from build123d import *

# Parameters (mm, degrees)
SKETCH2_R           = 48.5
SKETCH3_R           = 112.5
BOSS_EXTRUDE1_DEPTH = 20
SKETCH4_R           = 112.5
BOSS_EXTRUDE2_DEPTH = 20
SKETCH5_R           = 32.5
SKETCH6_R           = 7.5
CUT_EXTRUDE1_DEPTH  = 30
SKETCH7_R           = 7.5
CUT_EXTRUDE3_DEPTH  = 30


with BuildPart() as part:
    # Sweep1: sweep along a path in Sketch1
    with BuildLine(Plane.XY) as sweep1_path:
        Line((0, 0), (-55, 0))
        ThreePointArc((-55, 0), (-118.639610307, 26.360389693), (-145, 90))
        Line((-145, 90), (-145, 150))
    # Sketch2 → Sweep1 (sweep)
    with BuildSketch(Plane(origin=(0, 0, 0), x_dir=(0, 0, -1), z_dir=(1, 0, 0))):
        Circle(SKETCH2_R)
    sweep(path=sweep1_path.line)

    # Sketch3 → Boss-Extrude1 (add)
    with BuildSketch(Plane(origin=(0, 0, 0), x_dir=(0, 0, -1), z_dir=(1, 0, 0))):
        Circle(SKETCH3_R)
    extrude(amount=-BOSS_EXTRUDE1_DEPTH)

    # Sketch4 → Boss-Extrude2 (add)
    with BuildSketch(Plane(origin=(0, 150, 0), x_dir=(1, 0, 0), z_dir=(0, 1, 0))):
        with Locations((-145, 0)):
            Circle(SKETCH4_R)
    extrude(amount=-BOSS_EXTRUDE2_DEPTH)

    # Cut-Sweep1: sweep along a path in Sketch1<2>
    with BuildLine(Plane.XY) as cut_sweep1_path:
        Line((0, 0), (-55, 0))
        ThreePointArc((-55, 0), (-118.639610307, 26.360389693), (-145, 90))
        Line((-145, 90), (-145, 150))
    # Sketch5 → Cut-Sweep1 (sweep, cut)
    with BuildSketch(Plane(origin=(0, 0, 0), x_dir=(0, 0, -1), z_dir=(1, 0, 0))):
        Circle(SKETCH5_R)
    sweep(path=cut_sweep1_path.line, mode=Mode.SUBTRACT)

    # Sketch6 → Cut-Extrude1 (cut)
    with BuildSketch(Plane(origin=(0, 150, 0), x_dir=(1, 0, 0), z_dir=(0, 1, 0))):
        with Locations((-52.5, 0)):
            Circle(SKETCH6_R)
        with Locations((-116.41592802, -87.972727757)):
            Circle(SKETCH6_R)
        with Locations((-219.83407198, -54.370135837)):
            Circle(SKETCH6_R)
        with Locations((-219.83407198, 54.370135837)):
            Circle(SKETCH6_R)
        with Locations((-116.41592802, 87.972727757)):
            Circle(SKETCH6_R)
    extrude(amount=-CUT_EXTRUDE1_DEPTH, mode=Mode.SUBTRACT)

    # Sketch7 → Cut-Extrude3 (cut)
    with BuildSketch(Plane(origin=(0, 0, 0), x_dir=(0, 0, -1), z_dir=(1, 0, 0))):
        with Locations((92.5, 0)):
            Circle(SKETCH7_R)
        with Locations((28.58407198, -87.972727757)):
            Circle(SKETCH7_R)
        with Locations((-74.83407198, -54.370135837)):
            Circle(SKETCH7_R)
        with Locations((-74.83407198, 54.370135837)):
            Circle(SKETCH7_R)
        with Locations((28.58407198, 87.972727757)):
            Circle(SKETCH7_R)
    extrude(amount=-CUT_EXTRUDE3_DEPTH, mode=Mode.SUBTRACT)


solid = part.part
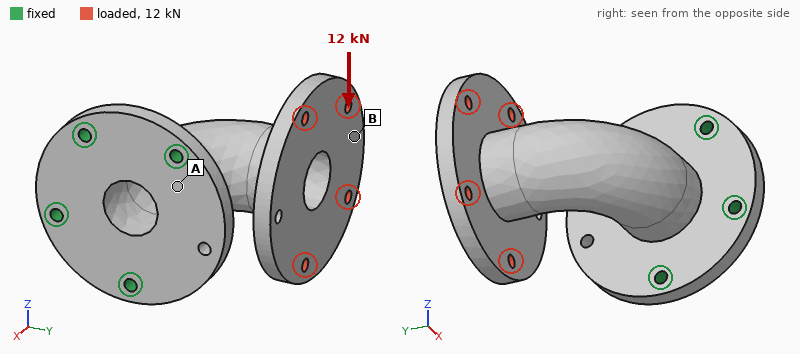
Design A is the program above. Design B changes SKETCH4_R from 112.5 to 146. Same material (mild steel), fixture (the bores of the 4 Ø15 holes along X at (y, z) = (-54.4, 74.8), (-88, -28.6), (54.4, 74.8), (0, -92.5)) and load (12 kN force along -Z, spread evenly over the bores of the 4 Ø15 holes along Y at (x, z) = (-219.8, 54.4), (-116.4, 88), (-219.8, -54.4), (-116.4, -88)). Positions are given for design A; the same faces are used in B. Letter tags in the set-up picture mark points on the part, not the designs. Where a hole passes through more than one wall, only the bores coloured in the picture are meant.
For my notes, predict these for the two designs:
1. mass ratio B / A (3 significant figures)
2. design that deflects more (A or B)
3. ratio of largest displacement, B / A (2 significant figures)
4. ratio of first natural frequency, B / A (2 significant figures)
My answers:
1.24
B
1.1
0.78
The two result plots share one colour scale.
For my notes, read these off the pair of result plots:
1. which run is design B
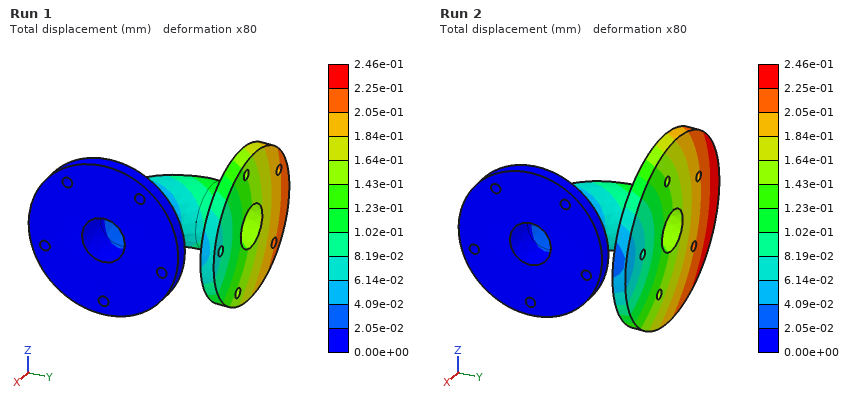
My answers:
Run 2
